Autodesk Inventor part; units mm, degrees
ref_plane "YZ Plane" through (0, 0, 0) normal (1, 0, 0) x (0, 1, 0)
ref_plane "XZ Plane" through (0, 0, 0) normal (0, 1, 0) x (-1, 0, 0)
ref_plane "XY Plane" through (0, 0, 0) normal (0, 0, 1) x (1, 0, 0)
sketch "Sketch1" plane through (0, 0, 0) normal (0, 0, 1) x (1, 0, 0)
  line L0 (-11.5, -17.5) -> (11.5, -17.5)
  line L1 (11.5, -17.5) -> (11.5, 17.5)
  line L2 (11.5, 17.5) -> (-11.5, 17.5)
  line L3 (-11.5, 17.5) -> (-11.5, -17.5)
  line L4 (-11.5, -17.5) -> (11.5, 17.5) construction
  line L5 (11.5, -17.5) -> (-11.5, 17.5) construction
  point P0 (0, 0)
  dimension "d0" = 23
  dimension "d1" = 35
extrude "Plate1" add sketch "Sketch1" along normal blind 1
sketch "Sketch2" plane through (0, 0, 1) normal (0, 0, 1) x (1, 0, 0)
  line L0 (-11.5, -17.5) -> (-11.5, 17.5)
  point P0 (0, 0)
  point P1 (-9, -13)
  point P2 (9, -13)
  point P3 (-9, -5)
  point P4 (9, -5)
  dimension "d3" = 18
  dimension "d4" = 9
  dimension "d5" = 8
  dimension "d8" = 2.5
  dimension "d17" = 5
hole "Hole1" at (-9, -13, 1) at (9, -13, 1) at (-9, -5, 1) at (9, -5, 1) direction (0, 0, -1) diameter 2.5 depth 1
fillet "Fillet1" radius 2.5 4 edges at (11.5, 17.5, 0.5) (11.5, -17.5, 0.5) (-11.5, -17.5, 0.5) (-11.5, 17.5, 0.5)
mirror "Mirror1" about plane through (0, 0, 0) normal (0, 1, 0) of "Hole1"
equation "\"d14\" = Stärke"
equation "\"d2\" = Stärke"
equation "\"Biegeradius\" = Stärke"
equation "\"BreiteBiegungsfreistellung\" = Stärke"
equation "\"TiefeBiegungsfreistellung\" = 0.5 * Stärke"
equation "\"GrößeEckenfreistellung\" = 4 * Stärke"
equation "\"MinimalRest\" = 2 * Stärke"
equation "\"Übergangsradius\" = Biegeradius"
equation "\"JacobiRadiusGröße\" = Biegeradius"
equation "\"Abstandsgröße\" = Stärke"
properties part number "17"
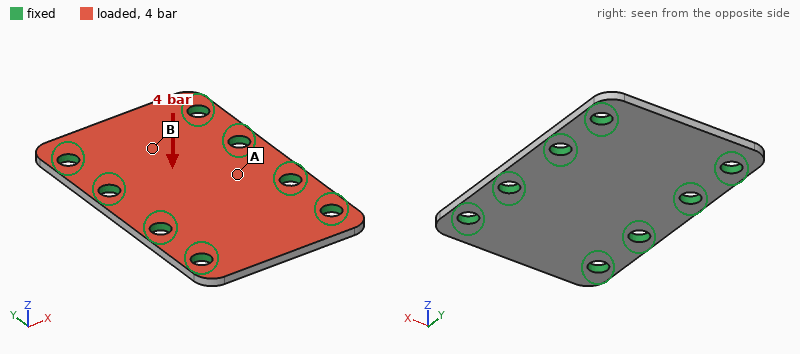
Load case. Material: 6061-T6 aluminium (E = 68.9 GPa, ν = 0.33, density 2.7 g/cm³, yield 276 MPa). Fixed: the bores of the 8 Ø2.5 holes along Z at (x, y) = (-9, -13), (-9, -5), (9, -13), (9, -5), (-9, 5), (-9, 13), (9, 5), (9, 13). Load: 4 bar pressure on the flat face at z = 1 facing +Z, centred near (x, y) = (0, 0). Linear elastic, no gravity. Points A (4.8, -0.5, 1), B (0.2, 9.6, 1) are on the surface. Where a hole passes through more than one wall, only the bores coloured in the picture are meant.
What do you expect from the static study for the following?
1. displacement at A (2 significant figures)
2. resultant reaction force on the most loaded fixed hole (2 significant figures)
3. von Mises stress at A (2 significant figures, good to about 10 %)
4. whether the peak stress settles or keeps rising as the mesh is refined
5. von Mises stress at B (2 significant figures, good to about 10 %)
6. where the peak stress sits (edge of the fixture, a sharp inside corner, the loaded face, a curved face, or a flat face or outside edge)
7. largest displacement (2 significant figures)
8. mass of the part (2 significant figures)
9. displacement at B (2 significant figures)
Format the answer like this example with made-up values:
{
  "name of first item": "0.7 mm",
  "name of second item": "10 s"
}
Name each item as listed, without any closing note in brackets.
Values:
{
  "displacement at A": "8.4 µm",
  "resultant reaction force on the most loaded fixed hole": "39 N",
  "von Mises stress at A": "8.3 MPa",
  "whether the peak stress settles or keeps rising as the mesh is refined": "keeps rising",
  "von Mises stress at B": "25 MPa",
  "where the peak stress sits": "edge of the fixture",
  "largest displacement": "18 µm",
  "mass of the part": "2.1 g",
  "displacement at B": "14 µm"
}
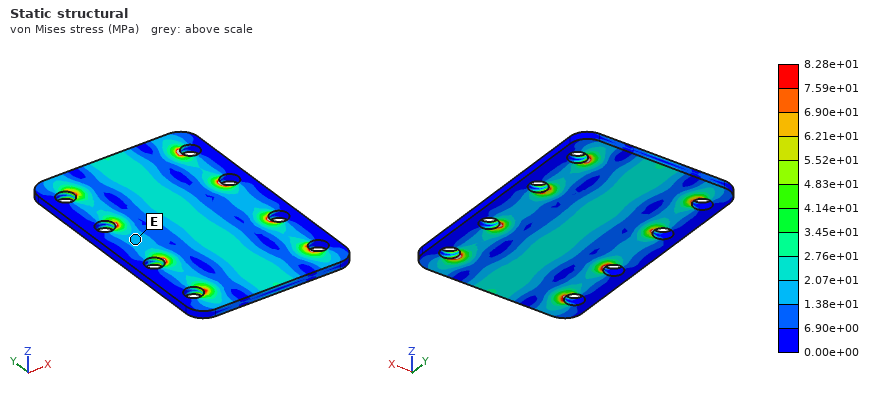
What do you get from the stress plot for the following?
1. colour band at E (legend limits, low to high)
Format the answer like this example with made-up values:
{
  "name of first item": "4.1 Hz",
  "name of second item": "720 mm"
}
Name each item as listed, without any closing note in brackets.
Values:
{
  "colour band at E": "1.38e+01 to 2.07e+01 MPa"
}
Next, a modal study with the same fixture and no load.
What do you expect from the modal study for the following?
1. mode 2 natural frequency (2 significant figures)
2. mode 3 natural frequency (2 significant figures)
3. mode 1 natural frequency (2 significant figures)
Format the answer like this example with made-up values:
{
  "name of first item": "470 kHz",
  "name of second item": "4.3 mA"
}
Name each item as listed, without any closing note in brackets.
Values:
{
  "mode 2 natural frequency": "19 kHz",
  "mode 3 natural frequency": "21 kHz",
  "mode 1 natural frequency": "18 kHz"
}
